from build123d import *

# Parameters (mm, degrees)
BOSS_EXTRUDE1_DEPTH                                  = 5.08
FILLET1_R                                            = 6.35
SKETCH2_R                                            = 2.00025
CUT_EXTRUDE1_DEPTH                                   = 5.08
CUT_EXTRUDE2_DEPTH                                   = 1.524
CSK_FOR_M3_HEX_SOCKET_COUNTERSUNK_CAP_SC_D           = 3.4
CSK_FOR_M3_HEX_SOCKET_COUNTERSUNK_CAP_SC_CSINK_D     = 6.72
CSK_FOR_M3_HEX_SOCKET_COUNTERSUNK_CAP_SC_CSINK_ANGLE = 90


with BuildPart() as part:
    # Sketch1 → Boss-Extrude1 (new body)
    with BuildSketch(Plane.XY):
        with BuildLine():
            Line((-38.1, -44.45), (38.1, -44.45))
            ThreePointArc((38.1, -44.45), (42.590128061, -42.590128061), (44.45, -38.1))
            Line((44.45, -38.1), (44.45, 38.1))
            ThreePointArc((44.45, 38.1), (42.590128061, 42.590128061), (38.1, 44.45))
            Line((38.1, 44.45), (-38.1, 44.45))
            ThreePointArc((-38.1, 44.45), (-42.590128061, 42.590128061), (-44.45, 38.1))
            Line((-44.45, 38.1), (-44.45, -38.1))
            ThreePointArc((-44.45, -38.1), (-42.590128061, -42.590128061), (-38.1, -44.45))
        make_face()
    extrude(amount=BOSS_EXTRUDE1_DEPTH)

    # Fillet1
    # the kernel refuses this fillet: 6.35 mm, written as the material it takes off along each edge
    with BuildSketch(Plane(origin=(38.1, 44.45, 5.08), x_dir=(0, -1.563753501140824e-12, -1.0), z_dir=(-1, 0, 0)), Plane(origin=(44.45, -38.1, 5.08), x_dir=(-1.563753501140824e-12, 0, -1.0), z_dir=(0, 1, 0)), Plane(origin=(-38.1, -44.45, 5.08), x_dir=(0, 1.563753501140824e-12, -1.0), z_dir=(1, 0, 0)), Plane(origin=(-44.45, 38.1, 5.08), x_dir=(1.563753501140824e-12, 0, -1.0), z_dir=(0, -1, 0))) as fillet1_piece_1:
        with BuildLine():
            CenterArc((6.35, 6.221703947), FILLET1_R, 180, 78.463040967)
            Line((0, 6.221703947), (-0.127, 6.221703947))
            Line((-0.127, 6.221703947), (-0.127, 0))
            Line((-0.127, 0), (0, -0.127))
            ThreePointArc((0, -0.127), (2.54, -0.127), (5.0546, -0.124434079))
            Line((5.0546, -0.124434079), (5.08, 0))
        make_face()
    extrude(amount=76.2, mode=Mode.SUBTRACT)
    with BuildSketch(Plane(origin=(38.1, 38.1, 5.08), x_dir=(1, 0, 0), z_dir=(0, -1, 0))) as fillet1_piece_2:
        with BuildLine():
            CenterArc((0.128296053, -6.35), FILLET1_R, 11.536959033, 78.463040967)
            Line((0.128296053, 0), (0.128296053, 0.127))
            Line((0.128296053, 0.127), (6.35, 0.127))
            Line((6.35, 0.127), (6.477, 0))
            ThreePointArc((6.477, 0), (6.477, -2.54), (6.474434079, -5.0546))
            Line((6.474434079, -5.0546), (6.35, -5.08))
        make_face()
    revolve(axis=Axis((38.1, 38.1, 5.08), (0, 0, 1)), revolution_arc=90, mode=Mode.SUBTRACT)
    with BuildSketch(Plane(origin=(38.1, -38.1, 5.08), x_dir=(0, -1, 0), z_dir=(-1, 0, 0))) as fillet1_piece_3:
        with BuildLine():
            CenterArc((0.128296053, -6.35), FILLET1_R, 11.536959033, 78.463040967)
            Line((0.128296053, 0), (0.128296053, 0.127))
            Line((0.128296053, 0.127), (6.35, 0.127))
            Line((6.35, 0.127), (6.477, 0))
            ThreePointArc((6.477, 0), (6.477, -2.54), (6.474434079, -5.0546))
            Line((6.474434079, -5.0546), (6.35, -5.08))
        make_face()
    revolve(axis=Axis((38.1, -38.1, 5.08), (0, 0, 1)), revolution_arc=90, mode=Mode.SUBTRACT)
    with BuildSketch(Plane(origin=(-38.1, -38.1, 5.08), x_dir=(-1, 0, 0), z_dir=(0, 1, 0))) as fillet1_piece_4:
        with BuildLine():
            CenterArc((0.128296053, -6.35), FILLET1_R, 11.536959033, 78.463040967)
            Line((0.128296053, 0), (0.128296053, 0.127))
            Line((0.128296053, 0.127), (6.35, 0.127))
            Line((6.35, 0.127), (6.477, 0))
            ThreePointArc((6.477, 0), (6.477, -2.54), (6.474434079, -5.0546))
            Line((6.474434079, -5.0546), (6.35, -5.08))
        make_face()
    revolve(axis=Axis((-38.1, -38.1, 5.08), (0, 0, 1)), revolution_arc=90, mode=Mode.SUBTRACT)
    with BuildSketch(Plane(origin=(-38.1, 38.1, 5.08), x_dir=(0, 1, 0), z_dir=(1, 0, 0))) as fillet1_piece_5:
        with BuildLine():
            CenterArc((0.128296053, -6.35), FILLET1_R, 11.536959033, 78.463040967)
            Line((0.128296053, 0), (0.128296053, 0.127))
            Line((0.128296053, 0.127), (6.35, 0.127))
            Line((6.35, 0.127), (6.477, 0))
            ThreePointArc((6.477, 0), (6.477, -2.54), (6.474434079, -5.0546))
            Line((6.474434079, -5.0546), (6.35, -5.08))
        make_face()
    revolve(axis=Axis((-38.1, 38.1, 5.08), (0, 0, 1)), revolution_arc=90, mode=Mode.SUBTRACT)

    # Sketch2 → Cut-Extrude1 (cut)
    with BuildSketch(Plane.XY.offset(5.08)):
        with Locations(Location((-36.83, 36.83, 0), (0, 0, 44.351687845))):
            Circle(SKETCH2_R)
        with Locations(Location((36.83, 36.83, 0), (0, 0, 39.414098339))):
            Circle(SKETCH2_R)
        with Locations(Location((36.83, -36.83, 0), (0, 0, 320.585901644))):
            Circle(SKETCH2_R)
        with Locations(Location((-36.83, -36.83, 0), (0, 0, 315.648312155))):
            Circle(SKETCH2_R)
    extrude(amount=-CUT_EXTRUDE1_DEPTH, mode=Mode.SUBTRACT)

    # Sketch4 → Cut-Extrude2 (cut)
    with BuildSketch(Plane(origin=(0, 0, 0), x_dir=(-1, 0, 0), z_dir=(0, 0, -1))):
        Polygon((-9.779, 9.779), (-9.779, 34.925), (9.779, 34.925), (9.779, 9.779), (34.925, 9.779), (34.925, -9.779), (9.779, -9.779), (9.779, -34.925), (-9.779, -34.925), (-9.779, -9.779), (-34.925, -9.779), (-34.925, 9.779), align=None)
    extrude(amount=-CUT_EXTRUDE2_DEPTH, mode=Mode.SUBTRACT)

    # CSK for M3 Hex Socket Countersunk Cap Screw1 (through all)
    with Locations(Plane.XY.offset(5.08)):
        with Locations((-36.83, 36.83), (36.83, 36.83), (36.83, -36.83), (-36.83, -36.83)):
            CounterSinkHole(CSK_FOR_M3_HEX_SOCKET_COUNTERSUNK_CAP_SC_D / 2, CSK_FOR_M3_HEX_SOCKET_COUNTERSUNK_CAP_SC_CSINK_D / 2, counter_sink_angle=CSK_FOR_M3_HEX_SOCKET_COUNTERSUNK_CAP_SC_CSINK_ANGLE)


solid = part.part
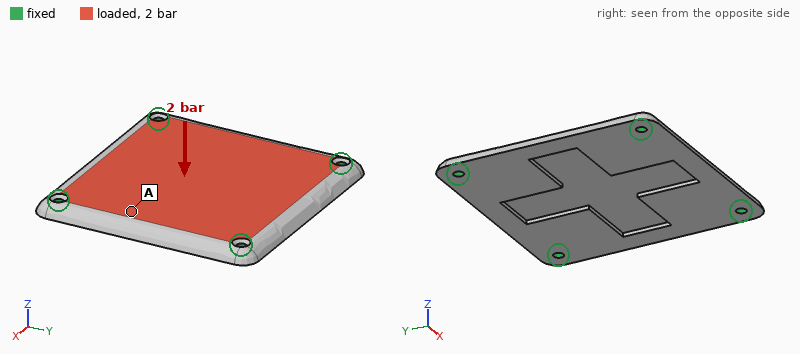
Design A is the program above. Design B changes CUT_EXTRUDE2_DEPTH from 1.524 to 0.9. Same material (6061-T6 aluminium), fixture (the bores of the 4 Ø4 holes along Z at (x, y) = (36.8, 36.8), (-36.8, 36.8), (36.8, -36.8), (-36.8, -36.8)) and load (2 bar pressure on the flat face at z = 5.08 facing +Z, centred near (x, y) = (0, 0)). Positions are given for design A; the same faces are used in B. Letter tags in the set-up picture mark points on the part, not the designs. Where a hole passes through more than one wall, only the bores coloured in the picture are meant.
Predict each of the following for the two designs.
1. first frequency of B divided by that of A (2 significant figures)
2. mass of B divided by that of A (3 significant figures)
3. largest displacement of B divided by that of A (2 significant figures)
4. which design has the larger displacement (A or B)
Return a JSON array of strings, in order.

["1.0", "1.04", "0.86", "A"]
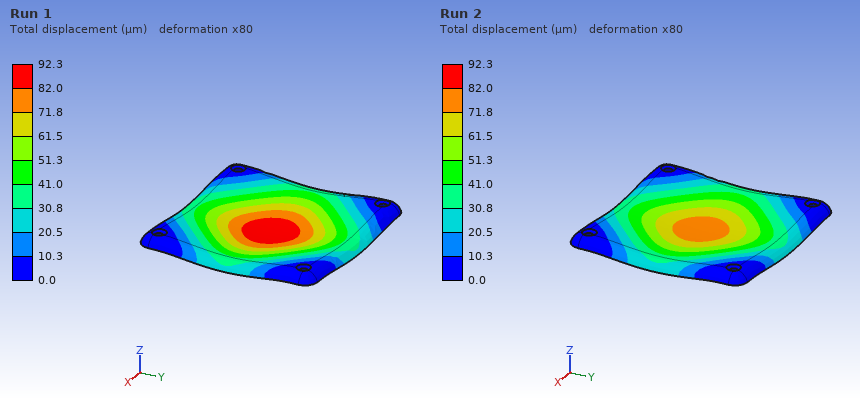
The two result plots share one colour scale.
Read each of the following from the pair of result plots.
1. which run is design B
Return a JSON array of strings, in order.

["Run 2"]
